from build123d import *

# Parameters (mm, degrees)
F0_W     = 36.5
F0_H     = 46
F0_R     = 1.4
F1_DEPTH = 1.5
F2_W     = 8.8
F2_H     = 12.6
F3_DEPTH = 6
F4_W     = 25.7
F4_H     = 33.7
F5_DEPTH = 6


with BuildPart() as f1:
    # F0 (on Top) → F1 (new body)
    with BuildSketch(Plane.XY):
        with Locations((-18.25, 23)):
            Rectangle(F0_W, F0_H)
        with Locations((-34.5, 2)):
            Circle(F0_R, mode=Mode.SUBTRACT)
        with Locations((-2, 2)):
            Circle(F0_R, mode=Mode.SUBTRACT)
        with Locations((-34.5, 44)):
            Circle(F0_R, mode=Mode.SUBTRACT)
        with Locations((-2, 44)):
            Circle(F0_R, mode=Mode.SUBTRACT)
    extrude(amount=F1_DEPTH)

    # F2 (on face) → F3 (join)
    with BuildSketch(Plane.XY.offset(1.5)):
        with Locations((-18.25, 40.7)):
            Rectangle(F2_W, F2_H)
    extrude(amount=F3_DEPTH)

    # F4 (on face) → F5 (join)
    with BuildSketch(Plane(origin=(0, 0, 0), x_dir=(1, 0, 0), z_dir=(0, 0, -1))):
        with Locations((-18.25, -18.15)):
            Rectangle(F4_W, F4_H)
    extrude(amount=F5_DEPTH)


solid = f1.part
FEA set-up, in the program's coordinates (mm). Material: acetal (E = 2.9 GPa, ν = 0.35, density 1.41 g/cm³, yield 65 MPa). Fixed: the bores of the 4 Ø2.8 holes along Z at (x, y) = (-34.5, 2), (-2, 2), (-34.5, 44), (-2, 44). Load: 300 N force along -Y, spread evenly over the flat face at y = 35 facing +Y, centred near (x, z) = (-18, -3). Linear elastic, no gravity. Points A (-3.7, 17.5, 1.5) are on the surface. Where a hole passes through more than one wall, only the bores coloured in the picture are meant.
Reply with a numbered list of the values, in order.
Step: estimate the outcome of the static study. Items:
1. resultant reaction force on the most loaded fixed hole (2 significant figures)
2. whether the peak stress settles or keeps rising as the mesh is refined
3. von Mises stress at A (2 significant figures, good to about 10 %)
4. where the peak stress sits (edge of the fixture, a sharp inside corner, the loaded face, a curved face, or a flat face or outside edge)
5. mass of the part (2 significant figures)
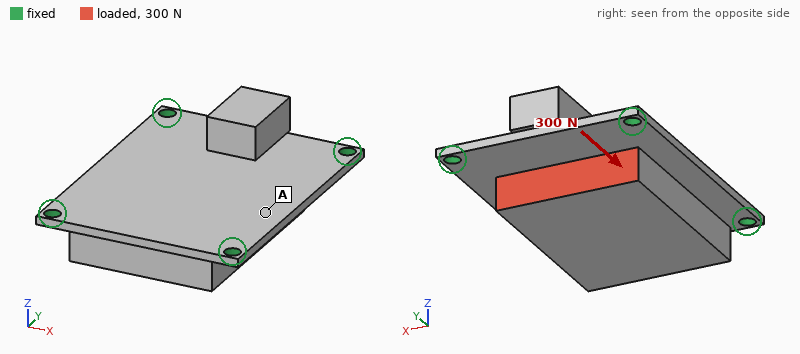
1. 88 N
2. keeps rising
3. 2.1 MPa
4. edge of the fixture
5. 12 g
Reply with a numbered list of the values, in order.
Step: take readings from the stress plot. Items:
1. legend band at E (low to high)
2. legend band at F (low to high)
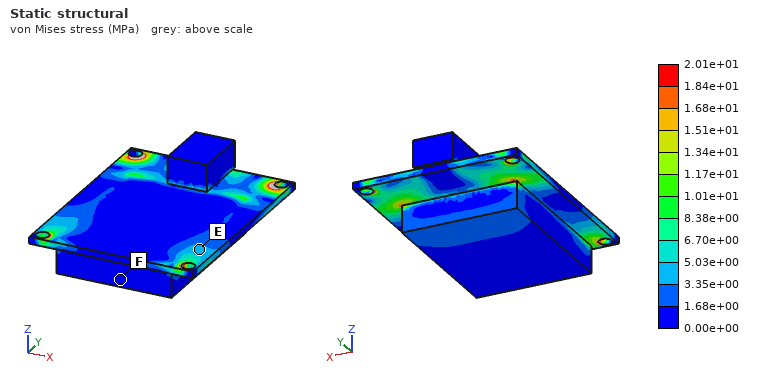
1. 3.35e+00 to 5.03e+00 MPa
2. 0.00e+00 to 1.68e+00 MPa
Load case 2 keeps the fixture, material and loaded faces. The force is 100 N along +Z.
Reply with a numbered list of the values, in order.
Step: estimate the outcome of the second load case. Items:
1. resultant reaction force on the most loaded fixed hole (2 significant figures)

1. 43 N
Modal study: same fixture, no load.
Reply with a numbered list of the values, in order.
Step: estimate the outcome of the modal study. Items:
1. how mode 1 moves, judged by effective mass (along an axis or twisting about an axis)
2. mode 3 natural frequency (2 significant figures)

1. along Z
2. 2700 Hz
